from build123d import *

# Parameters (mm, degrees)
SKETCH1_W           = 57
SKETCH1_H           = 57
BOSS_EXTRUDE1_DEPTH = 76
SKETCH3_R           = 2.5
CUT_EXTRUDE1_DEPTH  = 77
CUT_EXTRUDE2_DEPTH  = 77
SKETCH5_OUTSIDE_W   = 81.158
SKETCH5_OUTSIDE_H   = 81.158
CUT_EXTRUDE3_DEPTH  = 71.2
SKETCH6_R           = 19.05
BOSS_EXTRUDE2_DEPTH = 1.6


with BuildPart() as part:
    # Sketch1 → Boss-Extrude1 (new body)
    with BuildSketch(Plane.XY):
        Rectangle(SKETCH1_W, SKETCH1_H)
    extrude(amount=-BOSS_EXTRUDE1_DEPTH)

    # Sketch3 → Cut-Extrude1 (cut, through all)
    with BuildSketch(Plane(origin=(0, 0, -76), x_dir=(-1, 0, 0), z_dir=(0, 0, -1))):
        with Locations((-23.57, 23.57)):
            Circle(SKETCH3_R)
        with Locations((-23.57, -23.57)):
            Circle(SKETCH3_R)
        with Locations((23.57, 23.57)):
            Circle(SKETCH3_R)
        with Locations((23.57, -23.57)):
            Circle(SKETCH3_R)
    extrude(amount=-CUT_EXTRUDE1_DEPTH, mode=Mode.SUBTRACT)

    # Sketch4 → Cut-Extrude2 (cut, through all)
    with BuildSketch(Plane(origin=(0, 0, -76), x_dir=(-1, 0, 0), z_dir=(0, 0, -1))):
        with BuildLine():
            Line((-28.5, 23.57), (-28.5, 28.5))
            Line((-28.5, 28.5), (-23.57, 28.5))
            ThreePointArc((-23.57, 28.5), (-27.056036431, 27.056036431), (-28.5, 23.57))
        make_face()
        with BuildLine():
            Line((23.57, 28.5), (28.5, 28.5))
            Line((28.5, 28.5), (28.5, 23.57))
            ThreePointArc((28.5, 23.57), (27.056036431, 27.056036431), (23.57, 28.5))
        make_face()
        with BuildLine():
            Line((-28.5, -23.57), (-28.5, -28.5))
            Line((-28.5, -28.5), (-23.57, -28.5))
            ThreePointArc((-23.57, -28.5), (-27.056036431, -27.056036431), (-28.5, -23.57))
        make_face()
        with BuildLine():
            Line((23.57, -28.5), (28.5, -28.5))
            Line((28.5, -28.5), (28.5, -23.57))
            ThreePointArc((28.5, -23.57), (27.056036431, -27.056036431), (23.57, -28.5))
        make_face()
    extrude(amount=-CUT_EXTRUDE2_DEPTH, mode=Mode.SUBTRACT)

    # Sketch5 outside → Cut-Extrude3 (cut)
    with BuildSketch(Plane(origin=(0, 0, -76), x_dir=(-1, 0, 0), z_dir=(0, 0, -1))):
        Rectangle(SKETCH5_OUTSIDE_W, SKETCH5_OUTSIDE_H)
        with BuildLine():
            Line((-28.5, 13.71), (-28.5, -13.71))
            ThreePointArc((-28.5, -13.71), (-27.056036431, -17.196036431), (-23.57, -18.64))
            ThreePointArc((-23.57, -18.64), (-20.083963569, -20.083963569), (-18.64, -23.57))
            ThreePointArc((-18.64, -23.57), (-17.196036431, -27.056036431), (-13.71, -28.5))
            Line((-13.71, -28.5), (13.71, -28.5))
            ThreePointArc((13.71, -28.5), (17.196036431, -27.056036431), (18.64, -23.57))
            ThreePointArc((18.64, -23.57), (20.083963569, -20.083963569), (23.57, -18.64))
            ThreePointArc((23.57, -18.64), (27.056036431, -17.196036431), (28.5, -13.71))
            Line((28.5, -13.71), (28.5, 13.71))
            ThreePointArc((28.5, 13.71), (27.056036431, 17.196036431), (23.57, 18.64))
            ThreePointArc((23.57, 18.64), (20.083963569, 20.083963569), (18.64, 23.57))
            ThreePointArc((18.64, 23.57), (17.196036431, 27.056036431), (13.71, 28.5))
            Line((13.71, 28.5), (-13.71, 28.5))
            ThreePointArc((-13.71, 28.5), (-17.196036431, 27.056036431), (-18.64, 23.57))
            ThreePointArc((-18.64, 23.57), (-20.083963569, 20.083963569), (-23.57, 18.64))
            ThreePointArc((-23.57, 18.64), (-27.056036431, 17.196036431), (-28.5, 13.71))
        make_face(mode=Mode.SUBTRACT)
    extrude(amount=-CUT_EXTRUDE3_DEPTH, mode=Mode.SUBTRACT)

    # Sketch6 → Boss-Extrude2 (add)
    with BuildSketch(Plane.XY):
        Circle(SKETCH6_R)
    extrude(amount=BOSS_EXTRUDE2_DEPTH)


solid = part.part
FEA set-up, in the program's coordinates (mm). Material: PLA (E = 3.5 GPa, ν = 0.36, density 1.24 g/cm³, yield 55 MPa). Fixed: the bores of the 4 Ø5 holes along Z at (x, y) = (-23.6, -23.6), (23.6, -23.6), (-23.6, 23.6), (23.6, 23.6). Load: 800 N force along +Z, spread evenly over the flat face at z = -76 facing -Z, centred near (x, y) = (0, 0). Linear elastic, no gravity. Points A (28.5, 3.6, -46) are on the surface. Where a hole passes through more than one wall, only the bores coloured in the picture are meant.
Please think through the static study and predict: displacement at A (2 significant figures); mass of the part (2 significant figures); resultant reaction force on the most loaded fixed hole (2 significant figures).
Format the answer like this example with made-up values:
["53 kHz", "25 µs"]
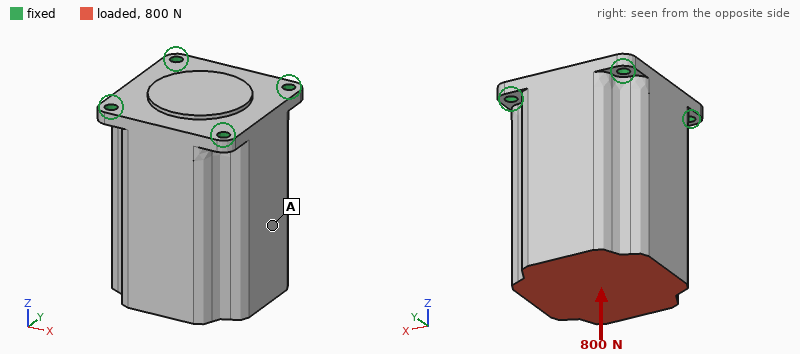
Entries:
["21 µm", "270 g", "220 N"]
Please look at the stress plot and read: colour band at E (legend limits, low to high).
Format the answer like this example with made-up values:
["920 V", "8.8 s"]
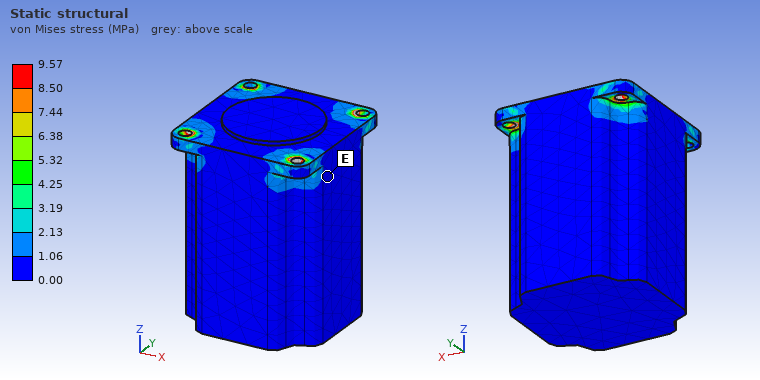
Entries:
["0.00 to 1.06 MPa"]
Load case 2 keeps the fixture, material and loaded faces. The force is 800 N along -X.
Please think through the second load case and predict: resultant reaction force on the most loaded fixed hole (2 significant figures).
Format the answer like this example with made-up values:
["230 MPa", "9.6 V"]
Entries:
["730 N"]
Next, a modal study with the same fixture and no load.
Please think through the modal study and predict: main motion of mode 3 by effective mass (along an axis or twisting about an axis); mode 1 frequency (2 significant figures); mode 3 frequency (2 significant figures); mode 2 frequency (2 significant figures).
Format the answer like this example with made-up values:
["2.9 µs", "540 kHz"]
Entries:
["along Z", "920 Hz", "1900 Hz", "920 Hz"]
